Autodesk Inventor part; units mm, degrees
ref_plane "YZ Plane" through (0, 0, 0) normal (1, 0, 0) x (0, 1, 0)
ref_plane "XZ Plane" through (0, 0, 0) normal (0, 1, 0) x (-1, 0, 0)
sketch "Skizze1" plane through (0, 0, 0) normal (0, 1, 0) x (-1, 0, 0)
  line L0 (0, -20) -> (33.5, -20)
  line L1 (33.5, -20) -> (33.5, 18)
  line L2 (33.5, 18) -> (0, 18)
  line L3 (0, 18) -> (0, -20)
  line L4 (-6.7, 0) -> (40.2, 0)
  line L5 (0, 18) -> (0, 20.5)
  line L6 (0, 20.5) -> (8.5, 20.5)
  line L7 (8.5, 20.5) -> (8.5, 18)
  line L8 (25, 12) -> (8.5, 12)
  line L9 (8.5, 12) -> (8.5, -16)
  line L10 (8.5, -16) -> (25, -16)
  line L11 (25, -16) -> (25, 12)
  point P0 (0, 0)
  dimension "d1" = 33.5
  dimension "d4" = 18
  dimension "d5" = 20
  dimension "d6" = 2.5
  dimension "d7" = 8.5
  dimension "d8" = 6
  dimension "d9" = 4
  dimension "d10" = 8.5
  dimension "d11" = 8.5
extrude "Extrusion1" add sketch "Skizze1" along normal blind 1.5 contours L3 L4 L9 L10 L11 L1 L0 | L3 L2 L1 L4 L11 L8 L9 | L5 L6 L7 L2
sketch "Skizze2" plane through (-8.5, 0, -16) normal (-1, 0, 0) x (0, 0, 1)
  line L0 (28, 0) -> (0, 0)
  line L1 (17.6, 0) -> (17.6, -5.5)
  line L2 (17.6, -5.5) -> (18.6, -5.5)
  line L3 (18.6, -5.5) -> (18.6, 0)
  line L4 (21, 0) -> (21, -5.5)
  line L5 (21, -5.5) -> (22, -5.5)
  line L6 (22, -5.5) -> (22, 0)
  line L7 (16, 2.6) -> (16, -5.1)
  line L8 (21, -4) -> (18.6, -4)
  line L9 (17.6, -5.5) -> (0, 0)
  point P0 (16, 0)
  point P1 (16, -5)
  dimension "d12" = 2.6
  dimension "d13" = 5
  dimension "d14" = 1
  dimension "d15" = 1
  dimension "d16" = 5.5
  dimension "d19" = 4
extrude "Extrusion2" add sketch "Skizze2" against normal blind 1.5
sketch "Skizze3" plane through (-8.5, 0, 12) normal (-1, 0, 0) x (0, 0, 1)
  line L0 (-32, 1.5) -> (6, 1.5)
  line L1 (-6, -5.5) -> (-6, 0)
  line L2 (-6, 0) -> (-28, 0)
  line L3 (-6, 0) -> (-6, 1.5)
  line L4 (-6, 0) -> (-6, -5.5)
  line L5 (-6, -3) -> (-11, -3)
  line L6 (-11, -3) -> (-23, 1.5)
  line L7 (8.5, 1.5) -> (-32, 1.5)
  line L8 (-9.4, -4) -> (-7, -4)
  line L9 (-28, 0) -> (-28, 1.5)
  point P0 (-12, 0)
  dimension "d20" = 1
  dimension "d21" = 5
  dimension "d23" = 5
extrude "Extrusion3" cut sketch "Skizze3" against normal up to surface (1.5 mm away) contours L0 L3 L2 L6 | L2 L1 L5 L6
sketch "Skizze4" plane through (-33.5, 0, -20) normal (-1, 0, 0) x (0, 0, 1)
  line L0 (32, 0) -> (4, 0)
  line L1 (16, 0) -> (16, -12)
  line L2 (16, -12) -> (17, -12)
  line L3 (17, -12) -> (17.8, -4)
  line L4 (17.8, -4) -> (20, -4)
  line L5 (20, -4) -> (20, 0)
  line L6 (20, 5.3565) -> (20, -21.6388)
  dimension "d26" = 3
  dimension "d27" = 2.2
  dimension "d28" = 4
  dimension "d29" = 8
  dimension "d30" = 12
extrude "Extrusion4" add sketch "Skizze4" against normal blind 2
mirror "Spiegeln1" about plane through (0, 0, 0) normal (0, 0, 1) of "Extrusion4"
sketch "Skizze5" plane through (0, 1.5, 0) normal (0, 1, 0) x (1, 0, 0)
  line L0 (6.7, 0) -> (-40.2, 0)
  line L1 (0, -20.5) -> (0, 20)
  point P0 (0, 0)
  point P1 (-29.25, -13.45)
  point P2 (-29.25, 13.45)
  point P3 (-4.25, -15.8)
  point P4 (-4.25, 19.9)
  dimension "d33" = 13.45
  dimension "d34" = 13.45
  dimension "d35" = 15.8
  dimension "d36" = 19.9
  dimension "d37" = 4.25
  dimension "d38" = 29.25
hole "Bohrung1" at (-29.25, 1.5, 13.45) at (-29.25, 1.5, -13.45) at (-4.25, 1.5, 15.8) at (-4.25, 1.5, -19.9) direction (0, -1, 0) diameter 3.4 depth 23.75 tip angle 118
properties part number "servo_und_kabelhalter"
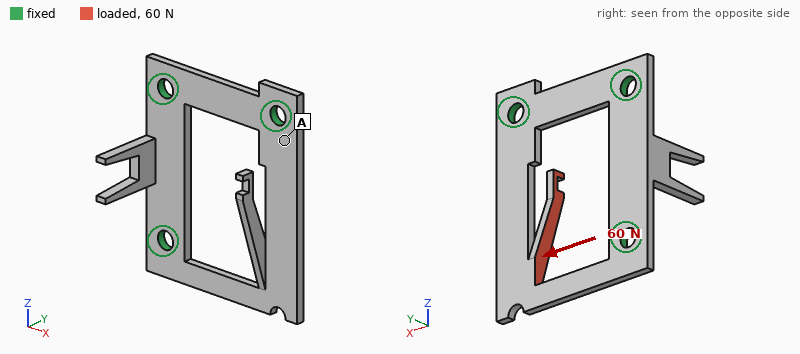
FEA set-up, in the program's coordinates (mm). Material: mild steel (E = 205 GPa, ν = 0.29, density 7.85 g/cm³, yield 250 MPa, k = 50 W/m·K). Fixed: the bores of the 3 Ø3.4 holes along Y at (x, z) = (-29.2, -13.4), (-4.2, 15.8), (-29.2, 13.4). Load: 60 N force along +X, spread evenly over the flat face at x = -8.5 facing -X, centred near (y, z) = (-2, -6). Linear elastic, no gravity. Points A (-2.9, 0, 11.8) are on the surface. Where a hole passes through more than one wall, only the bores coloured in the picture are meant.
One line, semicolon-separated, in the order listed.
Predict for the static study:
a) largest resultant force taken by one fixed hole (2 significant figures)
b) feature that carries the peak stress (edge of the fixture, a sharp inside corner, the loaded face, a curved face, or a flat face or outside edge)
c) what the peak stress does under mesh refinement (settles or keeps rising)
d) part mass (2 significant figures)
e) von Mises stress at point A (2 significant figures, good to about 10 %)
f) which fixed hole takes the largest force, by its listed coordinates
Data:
32 N; a sharp inside corner; keeps rising; 11 g; 29 MPa; (-29.2, -13.4)
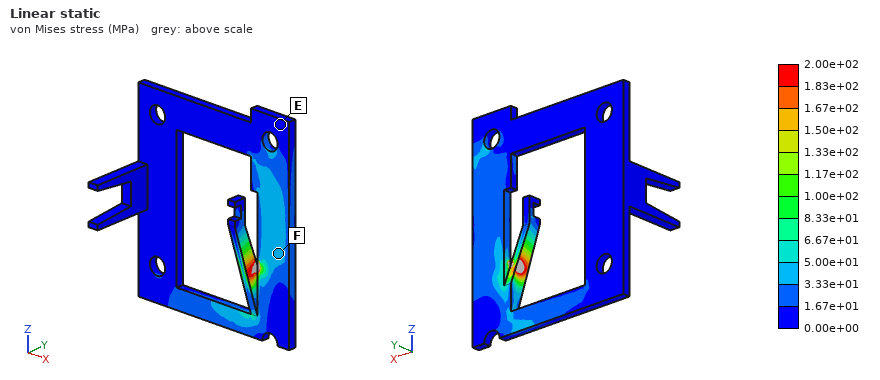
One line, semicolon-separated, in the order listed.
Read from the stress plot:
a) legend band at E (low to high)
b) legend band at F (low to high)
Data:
0.00e+00 to 1.67e+01 MPa; 3.33e+01 to 5.00e+01 MPa
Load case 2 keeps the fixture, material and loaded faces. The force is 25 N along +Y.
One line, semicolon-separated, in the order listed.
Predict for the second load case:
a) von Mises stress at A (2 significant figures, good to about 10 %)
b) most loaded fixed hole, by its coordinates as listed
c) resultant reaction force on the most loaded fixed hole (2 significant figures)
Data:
48 MPa; (-4.2, 15.8); 16 N
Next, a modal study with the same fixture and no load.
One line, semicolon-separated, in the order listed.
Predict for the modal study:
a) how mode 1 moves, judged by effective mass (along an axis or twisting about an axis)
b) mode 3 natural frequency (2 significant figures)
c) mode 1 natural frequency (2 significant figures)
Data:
along Y; 5400 Hz; 1800 Hz
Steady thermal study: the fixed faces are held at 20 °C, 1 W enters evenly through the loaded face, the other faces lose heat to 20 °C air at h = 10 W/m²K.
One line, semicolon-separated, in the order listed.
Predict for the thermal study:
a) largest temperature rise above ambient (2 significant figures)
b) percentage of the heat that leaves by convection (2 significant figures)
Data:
54 K; 16 %
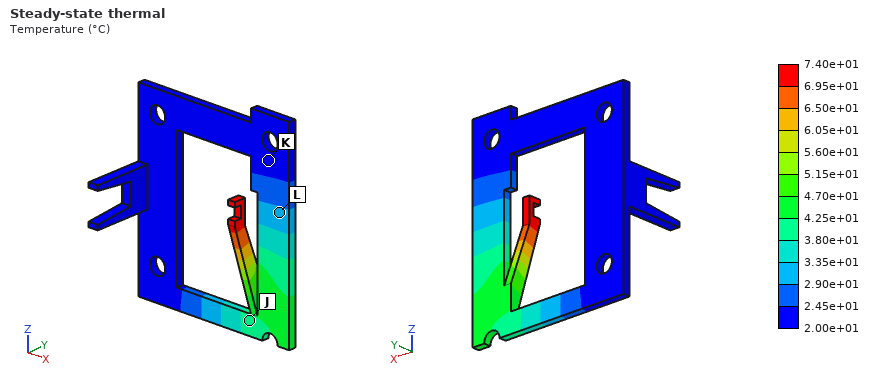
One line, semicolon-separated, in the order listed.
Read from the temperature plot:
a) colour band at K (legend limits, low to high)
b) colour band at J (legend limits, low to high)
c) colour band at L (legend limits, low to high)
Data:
2.00e+01 to 2.45e+01 °C; 3.80e+01 to 4.25e+01 °C; 2.90e+01 to 3.35e+01 °C
